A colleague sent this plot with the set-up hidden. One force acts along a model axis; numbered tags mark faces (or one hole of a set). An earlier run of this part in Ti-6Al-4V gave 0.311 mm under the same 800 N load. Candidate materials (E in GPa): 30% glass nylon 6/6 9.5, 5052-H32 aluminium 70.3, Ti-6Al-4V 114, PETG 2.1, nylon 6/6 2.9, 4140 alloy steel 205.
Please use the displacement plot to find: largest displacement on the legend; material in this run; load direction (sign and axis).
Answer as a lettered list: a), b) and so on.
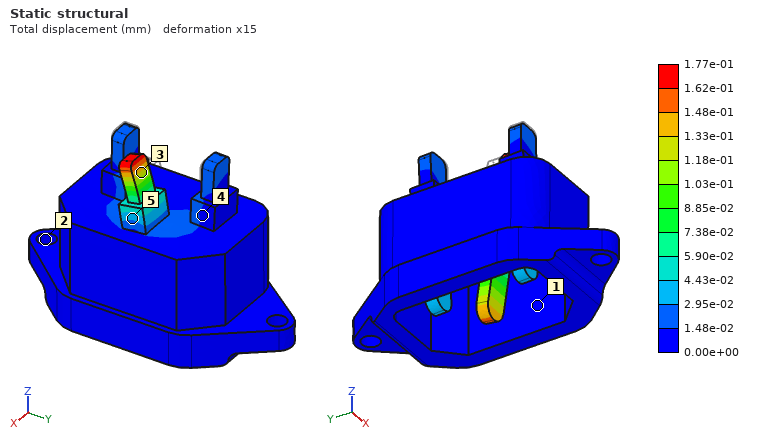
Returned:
a) 1.77e-01 mm
b) 4140 alloy steel
c) -Y
